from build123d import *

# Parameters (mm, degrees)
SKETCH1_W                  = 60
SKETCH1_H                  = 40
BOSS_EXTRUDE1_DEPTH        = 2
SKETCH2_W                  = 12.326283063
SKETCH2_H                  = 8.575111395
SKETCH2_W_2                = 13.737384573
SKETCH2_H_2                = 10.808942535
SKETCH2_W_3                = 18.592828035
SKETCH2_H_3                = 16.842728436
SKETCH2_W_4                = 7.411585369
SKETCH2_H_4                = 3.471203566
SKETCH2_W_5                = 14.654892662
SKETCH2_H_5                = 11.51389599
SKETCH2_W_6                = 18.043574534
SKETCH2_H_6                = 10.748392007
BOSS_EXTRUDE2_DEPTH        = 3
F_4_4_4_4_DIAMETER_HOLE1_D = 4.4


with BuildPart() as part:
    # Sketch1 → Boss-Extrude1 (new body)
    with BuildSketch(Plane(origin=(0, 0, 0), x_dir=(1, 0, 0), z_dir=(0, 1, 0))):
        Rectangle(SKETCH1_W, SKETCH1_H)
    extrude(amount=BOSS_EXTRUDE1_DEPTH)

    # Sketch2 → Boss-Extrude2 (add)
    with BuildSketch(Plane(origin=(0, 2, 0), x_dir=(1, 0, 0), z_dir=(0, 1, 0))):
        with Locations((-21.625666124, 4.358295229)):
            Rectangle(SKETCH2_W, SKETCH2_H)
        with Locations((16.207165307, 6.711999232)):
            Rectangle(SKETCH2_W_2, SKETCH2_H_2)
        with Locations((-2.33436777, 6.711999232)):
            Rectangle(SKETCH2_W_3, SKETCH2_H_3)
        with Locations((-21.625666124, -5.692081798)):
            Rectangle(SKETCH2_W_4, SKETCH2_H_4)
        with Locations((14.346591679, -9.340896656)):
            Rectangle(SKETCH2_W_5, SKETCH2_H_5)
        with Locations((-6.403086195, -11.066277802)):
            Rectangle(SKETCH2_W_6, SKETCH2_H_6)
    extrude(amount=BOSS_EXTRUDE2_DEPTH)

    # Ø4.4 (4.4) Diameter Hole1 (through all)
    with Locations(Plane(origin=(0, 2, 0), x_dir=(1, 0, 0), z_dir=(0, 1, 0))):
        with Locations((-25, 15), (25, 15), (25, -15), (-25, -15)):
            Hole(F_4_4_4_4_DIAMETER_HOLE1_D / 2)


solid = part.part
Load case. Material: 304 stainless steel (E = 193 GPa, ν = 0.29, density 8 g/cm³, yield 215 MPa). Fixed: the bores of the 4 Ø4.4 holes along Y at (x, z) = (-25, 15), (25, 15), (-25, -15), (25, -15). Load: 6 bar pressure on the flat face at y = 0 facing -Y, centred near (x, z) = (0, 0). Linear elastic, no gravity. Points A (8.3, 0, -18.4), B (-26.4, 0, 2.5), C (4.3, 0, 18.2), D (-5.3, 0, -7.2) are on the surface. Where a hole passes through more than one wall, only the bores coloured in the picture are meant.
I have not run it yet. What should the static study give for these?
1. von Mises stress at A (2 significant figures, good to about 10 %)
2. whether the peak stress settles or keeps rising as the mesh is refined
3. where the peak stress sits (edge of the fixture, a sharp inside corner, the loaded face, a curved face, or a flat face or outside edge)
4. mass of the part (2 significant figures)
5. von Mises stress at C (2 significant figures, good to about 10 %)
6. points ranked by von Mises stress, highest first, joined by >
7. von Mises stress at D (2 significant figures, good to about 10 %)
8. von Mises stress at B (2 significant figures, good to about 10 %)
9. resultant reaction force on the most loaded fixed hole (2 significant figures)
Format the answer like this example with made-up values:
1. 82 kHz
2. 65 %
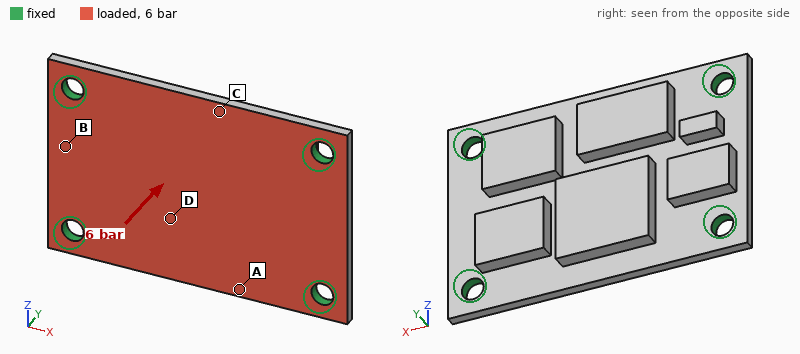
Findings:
1. 68 MPa
2. keeps rising
3. edge of the fixture
4. 60 g
5. 82 MPa
6. C > A > B > D
7. 17 MPa
8. 40 MPa
9. 410 N
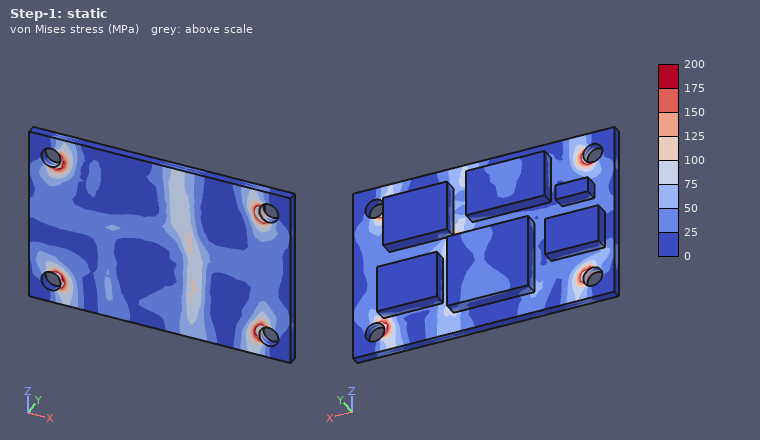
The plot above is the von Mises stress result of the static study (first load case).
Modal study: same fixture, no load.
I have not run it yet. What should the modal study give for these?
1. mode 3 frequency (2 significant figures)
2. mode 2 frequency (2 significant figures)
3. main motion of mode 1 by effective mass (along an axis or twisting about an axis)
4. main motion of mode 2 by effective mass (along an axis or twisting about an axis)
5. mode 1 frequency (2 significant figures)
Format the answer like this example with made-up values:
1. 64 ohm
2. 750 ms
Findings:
1. 10 kHz
2. 7000 Hz
3. along Y
4. twisting about X
5. 4000 Hz
